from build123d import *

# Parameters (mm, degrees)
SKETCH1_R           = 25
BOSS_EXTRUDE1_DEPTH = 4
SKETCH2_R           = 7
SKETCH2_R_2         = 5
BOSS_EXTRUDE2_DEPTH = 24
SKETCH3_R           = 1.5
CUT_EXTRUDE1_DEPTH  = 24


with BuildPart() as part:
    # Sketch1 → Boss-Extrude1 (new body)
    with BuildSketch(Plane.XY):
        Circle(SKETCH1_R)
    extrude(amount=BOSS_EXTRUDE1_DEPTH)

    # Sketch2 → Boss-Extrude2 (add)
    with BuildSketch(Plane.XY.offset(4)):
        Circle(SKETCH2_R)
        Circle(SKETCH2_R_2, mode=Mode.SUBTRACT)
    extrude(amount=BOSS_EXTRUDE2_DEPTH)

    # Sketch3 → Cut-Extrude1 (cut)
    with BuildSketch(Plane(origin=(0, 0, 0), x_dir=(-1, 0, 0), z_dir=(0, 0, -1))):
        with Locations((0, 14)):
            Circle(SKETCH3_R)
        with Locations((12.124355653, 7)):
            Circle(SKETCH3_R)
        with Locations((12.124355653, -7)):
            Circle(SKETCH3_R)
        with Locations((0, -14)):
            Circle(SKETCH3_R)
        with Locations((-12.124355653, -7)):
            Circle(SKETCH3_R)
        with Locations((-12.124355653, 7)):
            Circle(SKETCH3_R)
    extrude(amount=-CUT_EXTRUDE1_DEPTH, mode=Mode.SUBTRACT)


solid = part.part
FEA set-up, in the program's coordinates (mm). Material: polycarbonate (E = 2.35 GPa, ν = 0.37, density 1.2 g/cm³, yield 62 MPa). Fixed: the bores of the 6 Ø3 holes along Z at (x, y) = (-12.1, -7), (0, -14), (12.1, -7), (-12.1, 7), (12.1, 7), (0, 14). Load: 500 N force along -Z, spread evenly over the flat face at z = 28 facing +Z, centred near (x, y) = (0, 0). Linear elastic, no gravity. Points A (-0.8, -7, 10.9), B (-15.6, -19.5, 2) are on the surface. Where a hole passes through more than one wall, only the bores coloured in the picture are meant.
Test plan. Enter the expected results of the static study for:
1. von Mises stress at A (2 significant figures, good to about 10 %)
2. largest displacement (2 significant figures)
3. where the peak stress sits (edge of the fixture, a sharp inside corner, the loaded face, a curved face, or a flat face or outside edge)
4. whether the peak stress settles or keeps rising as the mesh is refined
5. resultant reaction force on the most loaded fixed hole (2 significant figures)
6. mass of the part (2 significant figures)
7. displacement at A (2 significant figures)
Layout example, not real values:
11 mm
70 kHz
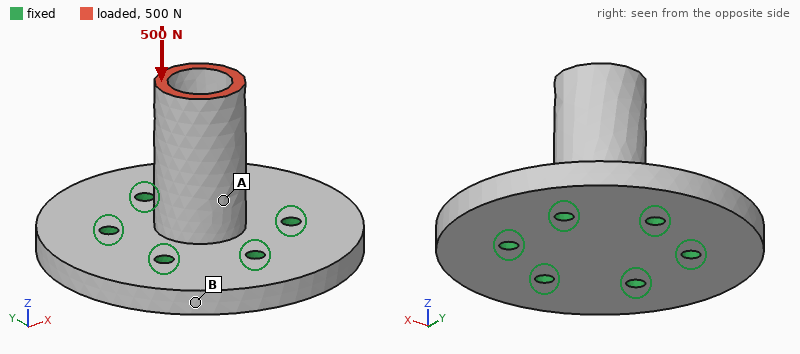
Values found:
5.8 MPa
0.12 mm
edge of the fixture
keeps rising
86 N
11 g
0.075 mm
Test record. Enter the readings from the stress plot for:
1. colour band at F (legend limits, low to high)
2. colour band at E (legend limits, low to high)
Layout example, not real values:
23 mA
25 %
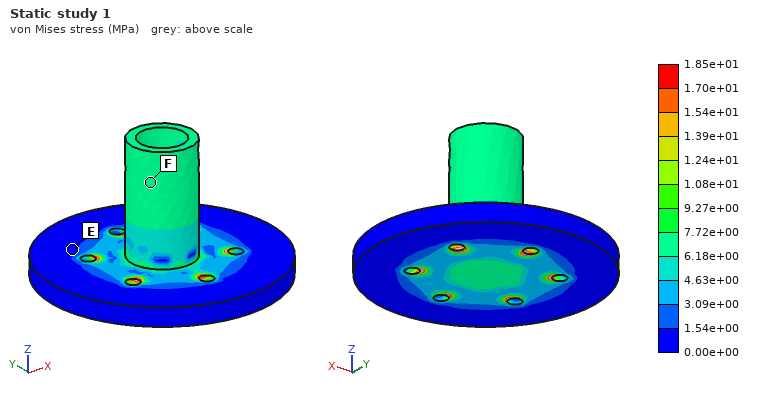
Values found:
6.18e+00 to 7.72e+00 MPa
0.00e+00 to 1.54e+00 MPa
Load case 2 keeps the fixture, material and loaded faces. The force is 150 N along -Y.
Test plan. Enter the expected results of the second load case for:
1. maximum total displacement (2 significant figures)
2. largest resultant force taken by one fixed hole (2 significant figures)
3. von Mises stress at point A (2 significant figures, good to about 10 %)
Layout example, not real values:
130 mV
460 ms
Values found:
0.54 mm
120 N
12 MPa
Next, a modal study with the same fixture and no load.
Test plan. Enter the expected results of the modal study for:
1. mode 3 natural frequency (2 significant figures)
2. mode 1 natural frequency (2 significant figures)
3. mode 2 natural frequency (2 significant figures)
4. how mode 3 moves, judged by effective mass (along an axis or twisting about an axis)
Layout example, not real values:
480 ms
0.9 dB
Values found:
6000 Hz
3200 Hz
3200 Hz
along Z
